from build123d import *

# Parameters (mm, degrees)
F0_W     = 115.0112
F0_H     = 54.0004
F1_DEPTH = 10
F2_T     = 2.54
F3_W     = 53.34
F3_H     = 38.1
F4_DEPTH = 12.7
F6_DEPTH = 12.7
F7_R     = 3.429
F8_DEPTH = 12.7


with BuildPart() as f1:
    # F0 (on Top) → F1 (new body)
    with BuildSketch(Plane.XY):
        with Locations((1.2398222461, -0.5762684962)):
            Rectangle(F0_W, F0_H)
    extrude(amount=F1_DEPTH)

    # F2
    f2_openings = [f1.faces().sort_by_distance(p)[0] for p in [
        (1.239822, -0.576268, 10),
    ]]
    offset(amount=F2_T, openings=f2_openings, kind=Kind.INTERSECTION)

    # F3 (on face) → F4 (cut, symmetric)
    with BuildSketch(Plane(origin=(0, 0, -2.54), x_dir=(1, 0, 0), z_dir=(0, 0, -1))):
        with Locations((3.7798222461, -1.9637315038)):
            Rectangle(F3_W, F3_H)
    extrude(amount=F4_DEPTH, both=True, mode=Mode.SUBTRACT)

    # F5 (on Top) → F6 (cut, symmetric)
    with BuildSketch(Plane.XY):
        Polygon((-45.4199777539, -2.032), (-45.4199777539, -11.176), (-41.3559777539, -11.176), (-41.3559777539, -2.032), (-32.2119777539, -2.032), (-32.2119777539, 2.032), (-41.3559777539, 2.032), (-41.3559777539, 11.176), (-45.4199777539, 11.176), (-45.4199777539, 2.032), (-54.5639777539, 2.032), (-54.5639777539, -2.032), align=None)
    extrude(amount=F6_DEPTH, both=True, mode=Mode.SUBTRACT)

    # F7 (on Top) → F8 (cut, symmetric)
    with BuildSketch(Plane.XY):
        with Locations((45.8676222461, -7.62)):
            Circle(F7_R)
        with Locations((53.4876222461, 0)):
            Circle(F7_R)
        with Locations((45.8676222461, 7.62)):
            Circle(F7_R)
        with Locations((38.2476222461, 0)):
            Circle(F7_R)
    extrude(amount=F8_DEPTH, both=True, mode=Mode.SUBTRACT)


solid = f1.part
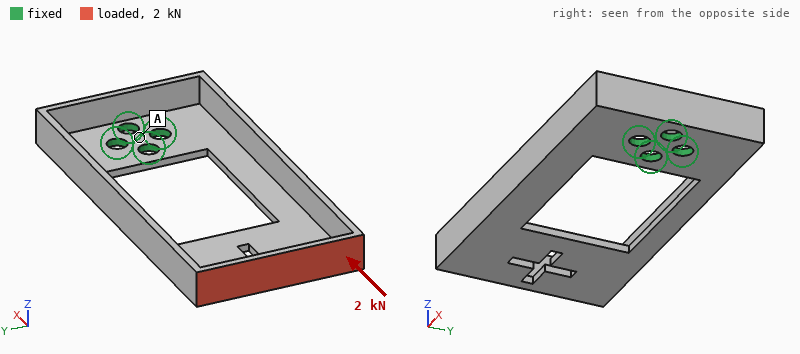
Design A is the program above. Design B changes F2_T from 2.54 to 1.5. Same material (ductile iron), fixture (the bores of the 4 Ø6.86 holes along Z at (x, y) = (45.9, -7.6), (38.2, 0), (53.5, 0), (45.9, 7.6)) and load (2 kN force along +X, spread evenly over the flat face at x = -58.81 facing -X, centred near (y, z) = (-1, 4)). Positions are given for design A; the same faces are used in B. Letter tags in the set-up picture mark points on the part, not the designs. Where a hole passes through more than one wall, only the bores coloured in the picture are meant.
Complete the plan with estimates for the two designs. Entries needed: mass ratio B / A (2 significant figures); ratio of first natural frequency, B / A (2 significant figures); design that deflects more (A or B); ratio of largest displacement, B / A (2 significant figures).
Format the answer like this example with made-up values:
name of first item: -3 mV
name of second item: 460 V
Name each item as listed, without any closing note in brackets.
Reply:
mass ratio B / A: 0.56
ratio of first natural frequency, B / A: 0.68
design that deflects more: B
ratio of largest displacement, B / A: 3.7
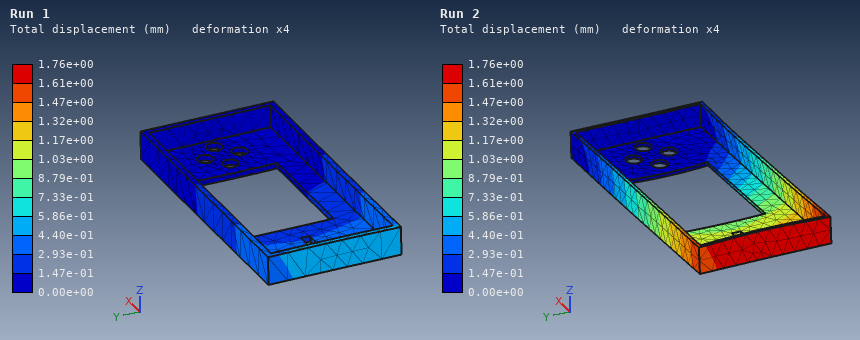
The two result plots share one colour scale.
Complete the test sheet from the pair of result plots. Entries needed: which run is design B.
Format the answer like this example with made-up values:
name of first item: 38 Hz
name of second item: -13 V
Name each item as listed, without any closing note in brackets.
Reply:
which run is design B: Run 2
